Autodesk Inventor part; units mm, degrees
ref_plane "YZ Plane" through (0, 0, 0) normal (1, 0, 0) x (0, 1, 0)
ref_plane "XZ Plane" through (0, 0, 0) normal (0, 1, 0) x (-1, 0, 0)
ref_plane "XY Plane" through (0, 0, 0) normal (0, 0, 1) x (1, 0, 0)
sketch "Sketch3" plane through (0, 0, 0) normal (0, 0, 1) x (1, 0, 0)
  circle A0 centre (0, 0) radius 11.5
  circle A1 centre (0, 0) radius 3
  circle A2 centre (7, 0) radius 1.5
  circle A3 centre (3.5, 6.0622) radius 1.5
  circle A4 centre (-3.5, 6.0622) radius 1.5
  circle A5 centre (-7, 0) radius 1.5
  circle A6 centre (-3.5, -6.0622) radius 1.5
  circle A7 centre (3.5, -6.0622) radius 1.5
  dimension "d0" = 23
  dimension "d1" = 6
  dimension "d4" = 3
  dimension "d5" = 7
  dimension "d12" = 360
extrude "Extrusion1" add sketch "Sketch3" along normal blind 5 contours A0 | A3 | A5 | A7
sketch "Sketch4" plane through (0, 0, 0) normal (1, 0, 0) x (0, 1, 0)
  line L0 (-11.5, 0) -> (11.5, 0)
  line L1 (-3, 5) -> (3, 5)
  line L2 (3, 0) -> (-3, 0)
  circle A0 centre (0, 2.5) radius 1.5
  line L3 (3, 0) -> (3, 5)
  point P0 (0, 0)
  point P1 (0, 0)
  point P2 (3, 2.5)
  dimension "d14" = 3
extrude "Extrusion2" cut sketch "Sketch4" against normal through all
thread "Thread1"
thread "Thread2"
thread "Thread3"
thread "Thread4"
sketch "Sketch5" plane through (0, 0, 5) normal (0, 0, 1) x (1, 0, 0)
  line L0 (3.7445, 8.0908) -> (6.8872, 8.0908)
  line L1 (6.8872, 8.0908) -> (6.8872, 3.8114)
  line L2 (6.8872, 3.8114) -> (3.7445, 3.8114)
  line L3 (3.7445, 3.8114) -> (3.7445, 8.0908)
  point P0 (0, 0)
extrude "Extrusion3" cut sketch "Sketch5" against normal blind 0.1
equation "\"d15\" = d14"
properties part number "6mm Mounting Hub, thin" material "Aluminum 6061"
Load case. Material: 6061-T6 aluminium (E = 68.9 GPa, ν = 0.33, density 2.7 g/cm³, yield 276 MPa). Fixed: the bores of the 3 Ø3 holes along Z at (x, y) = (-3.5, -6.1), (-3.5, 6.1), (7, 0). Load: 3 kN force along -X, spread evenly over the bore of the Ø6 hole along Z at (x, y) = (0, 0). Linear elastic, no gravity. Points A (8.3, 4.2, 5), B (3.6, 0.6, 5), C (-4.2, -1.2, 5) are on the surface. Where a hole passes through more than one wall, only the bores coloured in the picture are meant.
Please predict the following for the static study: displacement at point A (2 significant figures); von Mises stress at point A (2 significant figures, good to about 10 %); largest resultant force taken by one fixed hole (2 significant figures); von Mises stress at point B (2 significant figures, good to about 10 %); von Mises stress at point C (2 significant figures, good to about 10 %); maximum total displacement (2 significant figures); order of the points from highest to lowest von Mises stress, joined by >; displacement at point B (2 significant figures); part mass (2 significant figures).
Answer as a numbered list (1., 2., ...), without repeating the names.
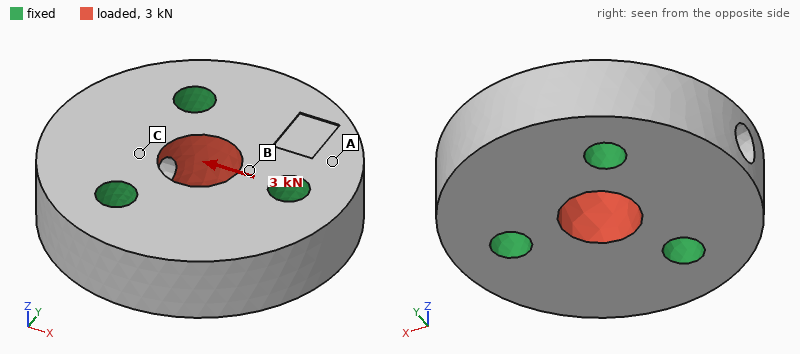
1. 0.70 µm
2. 8.9 MPa
3. 1.1 kN
4. 44 MPa
5. 30 MPa
6. 3.7 µm
7. B > C > A
8. 1.3 µm
9. 4.8 g
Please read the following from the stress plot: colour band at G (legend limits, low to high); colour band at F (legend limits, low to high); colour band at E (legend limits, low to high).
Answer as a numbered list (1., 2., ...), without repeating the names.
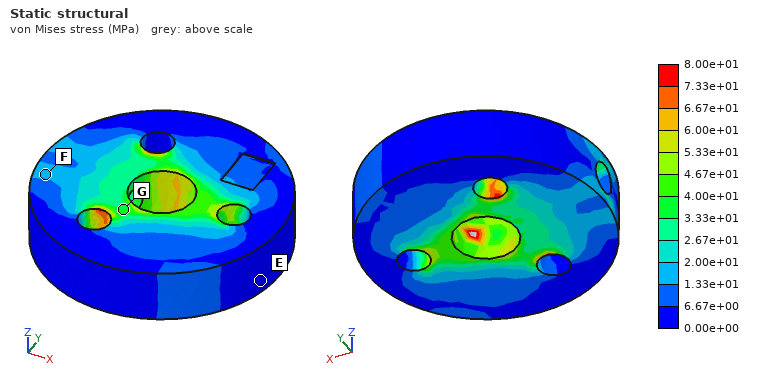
1. 3.33e+01 to 4.00e+01 MPa
2. 1.33e+01 to 2.00e+01 MPa
3. 0.00e+00 to 6.67e+00 MPa
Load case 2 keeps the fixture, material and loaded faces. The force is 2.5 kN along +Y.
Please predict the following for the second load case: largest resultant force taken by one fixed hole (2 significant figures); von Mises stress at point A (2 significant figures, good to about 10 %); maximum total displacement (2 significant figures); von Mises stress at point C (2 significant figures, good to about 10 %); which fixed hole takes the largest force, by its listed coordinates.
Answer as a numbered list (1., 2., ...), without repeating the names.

1. 930 N
2. 9.5 MPa
3. 3.1 µm
4. 20 MPa
5. (7, 0)
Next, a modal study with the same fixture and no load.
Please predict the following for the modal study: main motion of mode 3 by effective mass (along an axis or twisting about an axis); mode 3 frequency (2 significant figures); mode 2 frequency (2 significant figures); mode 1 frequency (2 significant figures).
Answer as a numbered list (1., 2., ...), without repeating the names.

1. along Z
2. 66 kHz
3. 60 kHz
4. 58 kHz
